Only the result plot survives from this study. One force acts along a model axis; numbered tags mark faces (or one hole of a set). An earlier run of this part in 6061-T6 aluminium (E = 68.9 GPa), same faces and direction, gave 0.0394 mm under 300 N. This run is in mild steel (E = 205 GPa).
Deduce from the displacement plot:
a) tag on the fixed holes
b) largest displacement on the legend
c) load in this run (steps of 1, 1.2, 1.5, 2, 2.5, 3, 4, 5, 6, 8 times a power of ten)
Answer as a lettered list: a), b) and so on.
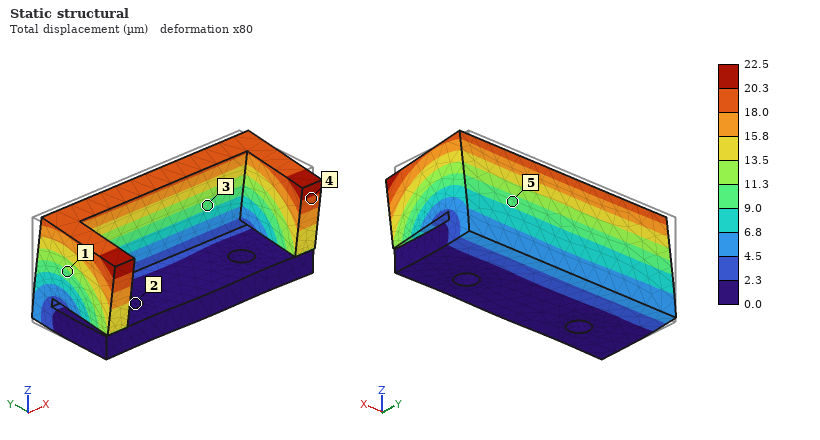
a) 2
b) 22.5 µm
c) 500 N
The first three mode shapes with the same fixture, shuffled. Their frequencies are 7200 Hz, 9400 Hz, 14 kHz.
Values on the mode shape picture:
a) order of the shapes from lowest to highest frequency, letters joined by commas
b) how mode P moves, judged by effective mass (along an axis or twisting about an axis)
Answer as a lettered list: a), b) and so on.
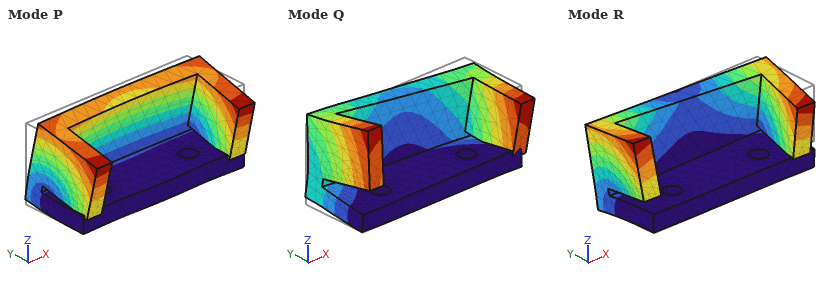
a) P, R, Q
b) along Y
